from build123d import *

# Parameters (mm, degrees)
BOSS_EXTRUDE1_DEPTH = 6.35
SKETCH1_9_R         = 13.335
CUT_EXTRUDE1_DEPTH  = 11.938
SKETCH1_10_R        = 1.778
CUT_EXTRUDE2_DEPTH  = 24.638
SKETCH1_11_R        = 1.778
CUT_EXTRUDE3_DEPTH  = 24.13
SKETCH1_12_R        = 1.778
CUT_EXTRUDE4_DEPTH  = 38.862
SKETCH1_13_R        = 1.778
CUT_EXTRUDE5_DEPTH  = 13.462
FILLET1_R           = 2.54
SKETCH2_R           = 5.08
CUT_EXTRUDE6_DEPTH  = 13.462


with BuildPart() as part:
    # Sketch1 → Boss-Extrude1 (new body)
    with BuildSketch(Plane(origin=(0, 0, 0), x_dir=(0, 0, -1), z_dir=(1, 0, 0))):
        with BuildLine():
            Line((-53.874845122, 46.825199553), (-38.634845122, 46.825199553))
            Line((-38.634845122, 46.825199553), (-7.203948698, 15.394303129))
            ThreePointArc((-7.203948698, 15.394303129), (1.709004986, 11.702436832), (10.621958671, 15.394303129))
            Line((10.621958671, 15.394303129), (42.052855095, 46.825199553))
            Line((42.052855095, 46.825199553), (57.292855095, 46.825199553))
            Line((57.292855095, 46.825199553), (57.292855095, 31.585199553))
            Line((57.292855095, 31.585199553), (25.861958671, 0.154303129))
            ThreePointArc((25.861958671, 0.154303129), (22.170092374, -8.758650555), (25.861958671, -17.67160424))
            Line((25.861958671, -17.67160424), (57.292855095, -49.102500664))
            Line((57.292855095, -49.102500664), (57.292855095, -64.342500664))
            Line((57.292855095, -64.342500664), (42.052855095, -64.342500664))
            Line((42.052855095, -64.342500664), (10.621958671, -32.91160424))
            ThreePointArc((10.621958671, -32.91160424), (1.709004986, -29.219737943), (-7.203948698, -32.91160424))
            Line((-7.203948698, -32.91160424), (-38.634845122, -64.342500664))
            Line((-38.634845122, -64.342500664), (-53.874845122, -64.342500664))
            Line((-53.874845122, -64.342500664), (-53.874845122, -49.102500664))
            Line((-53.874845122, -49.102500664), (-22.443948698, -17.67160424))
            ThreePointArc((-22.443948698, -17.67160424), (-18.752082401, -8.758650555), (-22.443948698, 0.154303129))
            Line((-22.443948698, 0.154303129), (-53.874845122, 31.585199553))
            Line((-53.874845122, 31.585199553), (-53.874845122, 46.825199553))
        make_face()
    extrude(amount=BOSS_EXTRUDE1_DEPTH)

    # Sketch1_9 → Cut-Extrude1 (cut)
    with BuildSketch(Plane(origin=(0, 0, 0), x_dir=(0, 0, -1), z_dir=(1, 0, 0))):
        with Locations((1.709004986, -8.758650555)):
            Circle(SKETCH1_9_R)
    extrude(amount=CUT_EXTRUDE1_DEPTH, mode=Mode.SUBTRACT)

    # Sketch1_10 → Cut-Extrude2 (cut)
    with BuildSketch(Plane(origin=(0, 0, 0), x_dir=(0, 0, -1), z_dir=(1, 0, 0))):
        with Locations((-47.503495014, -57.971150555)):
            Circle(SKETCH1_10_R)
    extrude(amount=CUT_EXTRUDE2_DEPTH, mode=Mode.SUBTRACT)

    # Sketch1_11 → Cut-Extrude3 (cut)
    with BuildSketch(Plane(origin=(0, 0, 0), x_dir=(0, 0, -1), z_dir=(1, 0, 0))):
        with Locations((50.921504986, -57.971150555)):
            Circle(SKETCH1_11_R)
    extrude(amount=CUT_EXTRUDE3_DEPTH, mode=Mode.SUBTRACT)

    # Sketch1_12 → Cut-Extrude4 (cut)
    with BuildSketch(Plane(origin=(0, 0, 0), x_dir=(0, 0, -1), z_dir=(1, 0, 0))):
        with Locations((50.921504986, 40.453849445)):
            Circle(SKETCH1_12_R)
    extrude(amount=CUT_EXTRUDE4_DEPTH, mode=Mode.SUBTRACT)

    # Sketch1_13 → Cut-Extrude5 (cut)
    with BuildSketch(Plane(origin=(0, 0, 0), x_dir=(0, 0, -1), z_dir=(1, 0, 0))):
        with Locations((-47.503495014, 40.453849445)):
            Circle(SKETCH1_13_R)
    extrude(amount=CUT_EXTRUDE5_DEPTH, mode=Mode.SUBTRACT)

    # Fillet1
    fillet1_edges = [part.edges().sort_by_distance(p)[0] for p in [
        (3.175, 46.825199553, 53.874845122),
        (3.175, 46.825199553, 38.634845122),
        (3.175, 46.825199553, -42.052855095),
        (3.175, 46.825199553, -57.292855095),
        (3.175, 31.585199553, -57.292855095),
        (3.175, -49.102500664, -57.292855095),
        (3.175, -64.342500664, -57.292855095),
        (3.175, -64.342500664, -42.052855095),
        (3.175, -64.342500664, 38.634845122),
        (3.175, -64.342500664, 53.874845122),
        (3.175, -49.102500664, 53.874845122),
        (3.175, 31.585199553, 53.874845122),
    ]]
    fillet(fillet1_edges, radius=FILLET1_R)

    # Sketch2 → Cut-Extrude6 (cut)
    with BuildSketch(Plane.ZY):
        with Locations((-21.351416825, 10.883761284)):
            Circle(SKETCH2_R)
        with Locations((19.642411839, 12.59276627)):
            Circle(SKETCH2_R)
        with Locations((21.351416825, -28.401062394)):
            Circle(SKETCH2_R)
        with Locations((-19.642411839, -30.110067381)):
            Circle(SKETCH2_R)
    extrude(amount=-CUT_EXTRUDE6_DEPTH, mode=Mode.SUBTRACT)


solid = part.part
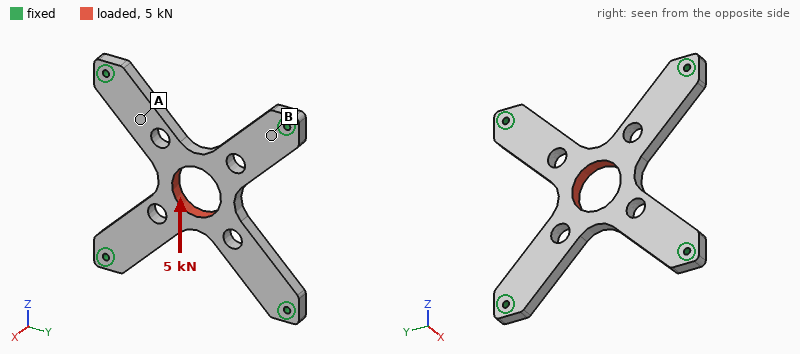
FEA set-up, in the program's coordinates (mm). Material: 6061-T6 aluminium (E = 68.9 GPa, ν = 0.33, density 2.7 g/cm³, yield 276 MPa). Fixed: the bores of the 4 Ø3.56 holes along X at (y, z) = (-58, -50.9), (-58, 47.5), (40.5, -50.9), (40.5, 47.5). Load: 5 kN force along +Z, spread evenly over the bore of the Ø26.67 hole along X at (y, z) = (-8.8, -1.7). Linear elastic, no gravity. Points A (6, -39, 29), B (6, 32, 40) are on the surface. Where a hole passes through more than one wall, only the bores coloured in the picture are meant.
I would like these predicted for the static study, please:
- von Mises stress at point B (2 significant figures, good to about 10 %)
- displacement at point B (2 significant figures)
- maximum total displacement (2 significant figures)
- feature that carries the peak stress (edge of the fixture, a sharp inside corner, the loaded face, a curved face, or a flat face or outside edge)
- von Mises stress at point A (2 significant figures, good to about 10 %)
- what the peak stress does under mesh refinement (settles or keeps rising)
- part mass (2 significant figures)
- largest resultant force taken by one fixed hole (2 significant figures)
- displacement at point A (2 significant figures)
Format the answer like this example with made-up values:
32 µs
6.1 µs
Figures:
17 MPa
4.7 µm
25 µm
edge of the fixture
9.8 MPa
keeps rising
87 g
1.7 kN
9.7 µm
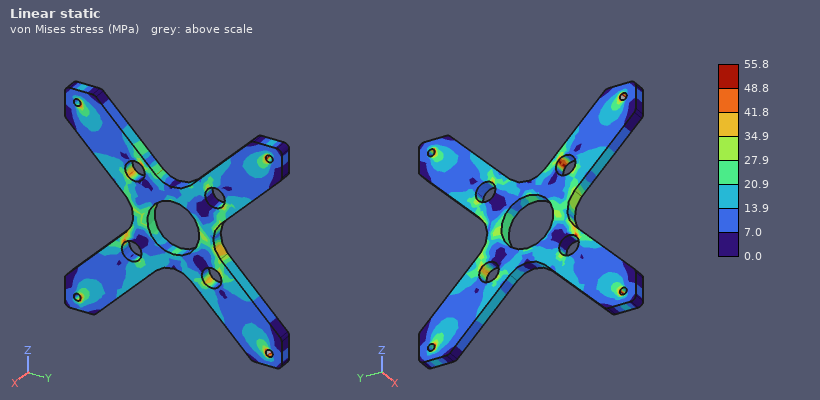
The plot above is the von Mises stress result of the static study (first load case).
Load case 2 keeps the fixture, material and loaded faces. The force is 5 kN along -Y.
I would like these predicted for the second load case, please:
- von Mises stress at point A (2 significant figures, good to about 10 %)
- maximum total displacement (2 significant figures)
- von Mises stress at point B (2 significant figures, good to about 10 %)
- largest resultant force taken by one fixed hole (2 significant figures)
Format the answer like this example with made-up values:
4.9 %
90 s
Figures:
8.2 MPa
25 µm
17 MPa
1.7 kN
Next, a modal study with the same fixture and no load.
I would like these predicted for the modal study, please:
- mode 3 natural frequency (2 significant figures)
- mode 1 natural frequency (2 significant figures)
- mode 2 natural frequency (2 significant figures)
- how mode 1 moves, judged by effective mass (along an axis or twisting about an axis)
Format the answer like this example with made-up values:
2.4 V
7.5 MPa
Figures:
4300 Hz
2000 Hz
4300 Hz
along X
